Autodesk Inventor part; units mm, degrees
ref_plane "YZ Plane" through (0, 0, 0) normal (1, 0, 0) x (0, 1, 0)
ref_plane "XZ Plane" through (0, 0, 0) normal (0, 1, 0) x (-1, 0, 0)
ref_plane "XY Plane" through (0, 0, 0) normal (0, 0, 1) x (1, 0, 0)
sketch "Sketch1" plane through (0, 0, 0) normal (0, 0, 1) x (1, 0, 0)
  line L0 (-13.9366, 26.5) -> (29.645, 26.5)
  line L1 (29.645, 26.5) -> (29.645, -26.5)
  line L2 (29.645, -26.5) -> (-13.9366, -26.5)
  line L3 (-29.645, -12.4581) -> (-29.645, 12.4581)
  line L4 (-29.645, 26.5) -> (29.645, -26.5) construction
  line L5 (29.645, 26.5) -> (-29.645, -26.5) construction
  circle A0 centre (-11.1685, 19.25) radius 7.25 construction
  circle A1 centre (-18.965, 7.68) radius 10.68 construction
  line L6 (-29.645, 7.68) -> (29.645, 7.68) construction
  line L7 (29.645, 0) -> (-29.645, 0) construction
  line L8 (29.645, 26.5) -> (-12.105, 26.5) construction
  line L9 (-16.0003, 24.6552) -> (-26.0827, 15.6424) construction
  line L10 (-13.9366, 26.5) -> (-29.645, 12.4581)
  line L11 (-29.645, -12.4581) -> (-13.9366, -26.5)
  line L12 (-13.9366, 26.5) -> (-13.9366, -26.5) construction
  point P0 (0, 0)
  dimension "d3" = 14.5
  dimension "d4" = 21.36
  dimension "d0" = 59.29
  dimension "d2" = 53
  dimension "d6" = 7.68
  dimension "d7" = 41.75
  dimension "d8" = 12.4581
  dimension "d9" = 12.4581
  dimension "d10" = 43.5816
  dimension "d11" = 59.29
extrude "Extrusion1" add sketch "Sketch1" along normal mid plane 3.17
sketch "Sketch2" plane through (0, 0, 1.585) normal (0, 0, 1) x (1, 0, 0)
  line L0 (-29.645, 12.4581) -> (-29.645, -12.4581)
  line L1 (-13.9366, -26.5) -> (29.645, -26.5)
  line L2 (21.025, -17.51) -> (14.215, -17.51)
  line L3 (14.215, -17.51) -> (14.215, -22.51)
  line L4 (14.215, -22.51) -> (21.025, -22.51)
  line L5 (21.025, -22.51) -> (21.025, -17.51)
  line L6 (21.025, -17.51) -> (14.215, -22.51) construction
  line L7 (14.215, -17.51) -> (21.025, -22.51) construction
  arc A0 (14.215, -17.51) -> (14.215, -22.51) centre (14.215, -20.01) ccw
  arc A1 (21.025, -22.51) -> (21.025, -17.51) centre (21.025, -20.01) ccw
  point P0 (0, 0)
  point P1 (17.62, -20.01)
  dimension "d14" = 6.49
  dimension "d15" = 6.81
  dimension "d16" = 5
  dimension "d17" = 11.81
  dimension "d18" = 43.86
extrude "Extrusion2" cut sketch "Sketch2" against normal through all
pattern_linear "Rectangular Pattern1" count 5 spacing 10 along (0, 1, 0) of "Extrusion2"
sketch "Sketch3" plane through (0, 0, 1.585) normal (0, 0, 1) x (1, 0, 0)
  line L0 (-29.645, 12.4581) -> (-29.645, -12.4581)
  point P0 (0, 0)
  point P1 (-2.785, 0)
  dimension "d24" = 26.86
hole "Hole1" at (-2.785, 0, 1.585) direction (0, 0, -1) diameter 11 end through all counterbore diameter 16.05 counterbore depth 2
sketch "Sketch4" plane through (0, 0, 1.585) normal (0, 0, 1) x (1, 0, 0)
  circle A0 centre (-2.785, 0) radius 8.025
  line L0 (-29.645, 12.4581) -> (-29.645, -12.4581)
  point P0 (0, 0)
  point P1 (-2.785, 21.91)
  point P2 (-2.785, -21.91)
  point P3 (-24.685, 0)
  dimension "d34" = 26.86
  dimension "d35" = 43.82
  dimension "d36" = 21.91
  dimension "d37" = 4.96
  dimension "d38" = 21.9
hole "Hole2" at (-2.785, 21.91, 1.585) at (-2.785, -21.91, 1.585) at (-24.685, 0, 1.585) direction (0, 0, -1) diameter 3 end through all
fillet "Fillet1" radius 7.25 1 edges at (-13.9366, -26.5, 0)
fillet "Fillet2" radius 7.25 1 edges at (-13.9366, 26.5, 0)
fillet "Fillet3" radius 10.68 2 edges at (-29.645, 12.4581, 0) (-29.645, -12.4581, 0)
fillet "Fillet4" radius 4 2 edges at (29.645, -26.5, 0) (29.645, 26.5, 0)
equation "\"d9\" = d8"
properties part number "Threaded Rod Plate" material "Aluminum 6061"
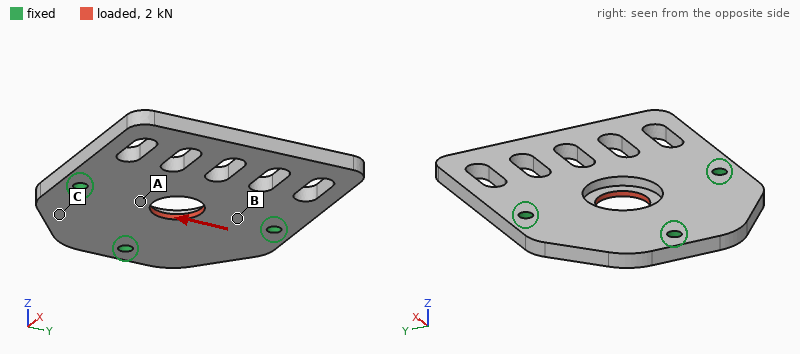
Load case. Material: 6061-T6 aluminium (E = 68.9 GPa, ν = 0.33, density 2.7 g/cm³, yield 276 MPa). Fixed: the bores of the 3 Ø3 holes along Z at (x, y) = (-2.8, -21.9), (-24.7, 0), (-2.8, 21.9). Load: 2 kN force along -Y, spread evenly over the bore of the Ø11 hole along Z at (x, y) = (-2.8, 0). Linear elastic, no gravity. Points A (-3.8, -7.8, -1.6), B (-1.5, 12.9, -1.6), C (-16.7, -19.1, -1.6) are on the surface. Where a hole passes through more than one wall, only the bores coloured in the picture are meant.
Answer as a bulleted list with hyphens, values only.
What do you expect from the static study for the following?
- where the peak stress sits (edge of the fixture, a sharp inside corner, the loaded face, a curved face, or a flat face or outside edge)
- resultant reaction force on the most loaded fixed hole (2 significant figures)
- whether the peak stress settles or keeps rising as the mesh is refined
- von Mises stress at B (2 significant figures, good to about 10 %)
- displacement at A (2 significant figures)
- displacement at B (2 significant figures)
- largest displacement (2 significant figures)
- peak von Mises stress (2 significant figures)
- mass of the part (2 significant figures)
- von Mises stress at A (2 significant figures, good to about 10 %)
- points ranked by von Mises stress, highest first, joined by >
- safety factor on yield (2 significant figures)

- the loaded face
- 830 N
- settles
- 33 MPa
- 7.1 µm
- 3.6 µm
- 10 µm
- 89 MPa
- 21 g
- 52 MPa
- A > B > C
- 3.1
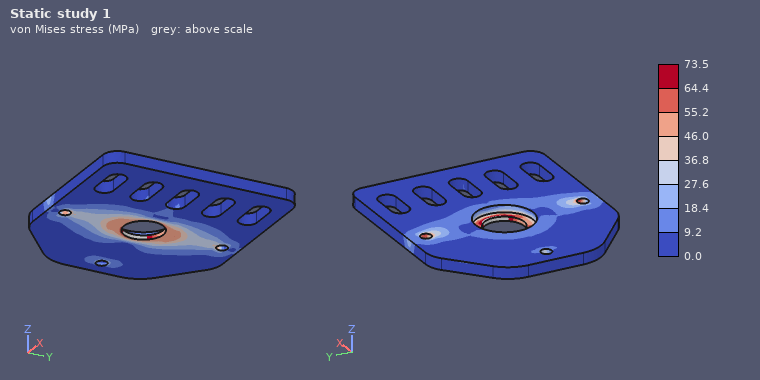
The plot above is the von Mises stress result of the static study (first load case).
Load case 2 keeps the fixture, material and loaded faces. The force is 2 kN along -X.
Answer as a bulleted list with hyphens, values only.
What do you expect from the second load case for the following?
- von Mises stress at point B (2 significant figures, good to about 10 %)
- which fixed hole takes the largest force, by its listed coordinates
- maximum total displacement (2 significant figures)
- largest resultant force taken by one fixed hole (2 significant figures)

- 13 MPa
- (-24.7, 0)
- 43 µm
- 800 N
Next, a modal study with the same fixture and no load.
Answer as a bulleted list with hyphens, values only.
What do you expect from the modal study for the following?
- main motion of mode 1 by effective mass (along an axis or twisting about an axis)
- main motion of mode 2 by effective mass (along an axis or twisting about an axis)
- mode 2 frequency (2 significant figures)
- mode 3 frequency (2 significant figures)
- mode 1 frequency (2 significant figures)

- along Z
- twisting about X
- 4100 Hz
- 7300 Hz
- 2100 Hz
